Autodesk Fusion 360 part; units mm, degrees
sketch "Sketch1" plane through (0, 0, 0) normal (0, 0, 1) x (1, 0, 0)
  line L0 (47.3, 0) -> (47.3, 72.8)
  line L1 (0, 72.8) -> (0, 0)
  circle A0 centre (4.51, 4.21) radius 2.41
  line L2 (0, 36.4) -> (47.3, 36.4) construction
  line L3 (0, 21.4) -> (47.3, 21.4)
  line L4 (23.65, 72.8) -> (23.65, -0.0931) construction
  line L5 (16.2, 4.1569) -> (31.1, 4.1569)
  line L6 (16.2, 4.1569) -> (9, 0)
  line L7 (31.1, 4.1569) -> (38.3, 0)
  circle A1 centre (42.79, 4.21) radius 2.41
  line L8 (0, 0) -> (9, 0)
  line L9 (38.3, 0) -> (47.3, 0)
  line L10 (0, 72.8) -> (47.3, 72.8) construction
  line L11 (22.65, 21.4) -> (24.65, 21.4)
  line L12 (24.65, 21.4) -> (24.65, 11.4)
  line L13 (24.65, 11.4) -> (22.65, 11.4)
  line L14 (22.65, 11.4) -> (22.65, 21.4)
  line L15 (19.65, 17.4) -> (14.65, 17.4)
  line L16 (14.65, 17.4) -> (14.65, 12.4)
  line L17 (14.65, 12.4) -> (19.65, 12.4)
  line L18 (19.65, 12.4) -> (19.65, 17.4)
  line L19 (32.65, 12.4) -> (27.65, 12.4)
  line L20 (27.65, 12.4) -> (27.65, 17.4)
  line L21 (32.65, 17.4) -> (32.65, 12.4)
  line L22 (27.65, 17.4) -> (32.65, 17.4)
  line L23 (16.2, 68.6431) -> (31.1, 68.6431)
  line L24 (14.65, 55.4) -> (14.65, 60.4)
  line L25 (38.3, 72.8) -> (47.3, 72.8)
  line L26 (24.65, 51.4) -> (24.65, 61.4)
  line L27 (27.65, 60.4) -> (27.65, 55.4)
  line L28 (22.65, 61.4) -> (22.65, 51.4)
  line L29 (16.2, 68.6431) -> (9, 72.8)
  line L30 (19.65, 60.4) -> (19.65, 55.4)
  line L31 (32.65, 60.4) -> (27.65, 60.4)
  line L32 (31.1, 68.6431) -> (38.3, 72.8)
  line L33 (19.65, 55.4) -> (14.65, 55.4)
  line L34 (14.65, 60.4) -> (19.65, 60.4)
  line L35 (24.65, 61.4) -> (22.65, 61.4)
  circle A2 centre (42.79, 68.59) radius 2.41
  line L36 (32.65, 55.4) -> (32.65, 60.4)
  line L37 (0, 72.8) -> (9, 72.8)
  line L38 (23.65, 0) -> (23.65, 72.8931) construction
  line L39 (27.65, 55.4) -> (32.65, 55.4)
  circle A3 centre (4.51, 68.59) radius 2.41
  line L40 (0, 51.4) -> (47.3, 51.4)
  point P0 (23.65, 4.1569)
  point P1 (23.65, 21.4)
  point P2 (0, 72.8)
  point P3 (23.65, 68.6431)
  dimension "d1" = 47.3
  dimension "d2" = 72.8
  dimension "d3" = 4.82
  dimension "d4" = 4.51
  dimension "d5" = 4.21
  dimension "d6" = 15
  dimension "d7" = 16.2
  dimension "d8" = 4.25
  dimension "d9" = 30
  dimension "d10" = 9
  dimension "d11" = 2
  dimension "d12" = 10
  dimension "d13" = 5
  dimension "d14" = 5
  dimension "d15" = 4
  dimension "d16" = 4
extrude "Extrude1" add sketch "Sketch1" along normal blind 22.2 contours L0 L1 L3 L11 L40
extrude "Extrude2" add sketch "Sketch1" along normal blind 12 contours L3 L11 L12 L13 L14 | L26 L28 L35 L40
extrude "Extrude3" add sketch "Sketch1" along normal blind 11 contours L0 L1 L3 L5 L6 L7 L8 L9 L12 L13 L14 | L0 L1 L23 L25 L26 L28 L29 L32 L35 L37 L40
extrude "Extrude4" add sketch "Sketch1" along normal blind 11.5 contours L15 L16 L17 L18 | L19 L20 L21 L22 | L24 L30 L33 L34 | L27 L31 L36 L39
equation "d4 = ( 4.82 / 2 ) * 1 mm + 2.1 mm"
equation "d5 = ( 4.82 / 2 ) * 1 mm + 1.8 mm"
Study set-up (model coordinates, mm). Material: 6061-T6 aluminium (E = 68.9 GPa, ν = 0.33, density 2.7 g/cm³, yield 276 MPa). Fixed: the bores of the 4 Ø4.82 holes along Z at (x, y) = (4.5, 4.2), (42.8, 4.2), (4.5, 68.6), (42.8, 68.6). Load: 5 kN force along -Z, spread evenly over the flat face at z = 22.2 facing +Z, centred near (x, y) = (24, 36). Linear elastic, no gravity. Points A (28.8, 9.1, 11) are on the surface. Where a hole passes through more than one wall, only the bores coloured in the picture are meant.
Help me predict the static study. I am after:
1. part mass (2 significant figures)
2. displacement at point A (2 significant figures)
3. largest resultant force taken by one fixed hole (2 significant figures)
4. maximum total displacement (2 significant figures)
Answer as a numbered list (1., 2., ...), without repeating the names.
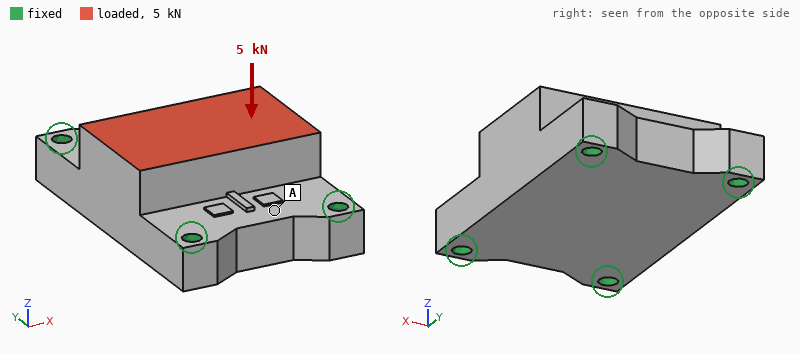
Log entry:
1. 140 g
2. 5.7 µm
3. 1.3 kN
4. 16 µm
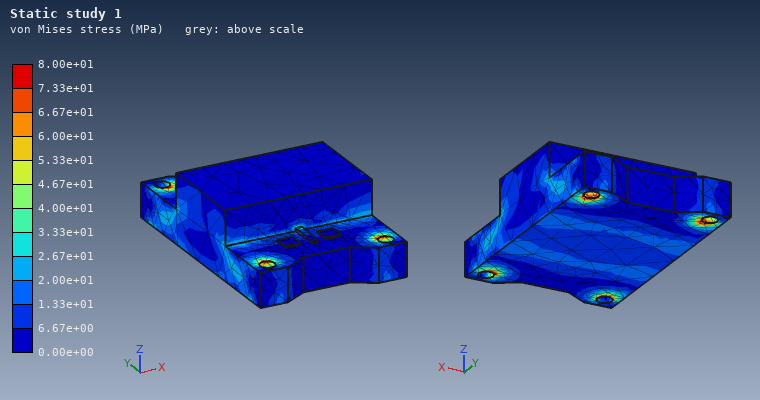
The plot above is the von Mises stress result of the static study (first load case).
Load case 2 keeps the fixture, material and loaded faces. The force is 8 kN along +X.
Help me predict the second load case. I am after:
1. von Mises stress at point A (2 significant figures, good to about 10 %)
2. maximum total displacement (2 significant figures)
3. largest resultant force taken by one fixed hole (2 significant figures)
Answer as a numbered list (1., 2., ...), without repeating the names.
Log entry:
1. 32 MPa
2. 44 µm
3. 3.2 kN
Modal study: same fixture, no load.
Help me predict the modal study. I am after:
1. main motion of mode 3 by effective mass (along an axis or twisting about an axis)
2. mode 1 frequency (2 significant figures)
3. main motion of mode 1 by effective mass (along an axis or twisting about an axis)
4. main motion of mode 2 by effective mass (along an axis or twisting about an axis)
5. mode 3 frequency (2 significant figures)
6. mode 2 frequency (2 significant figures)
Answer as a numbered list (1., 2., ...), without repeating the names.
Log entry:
1. along X
2. 9400 Hz
3. along Z
4. along X
5. 17 kHz
6. 11 kHz
